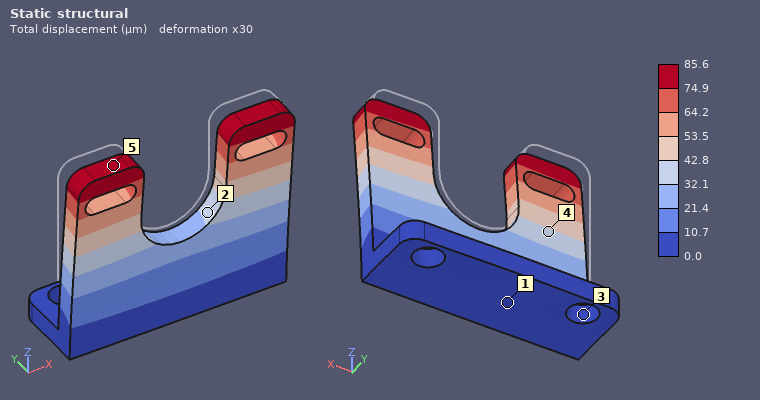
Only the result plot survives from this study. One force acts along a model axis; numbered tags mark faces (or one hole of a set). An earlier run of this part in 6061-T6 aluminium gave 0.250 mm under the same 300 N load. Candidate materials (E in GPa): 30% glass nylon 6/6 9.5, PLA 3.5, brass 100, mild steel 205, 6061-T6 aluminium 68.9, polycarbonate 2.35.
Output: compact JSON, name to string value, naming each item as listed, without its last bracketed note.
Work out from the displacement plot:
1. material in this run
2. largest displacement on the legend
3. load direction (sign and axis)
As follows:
{"material in this run": "mild steel", "largest displacement on the legend": "85.6 µm", "load direction": "-Y"}
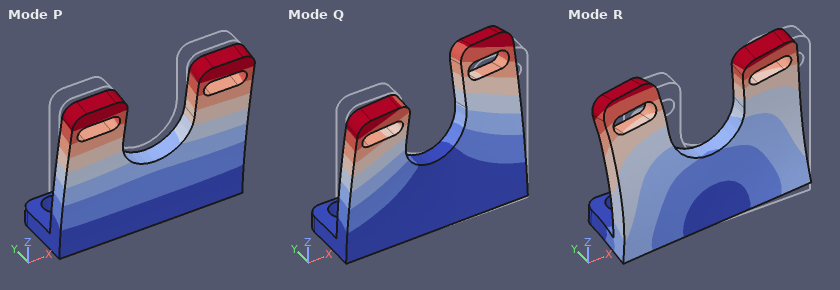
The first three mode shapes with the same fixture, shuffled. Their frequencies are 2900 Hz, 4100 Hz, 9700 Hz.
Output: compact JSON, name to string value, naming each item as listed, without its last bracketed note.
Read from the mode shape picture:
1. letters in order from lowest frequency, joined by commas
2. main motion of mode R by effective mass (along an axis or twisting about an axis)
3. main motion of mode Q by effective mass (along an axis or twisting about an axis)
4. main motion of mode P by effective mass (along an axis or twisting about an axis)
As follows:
{"letters in order from lowest frequency, joined by commas": "P, Q, R", "main motion of mode R by effective mass": "along X", "main motion of mode Q by effective mass": "twisting about Z", "main motion of mode P by effective mass": "along Y"}
